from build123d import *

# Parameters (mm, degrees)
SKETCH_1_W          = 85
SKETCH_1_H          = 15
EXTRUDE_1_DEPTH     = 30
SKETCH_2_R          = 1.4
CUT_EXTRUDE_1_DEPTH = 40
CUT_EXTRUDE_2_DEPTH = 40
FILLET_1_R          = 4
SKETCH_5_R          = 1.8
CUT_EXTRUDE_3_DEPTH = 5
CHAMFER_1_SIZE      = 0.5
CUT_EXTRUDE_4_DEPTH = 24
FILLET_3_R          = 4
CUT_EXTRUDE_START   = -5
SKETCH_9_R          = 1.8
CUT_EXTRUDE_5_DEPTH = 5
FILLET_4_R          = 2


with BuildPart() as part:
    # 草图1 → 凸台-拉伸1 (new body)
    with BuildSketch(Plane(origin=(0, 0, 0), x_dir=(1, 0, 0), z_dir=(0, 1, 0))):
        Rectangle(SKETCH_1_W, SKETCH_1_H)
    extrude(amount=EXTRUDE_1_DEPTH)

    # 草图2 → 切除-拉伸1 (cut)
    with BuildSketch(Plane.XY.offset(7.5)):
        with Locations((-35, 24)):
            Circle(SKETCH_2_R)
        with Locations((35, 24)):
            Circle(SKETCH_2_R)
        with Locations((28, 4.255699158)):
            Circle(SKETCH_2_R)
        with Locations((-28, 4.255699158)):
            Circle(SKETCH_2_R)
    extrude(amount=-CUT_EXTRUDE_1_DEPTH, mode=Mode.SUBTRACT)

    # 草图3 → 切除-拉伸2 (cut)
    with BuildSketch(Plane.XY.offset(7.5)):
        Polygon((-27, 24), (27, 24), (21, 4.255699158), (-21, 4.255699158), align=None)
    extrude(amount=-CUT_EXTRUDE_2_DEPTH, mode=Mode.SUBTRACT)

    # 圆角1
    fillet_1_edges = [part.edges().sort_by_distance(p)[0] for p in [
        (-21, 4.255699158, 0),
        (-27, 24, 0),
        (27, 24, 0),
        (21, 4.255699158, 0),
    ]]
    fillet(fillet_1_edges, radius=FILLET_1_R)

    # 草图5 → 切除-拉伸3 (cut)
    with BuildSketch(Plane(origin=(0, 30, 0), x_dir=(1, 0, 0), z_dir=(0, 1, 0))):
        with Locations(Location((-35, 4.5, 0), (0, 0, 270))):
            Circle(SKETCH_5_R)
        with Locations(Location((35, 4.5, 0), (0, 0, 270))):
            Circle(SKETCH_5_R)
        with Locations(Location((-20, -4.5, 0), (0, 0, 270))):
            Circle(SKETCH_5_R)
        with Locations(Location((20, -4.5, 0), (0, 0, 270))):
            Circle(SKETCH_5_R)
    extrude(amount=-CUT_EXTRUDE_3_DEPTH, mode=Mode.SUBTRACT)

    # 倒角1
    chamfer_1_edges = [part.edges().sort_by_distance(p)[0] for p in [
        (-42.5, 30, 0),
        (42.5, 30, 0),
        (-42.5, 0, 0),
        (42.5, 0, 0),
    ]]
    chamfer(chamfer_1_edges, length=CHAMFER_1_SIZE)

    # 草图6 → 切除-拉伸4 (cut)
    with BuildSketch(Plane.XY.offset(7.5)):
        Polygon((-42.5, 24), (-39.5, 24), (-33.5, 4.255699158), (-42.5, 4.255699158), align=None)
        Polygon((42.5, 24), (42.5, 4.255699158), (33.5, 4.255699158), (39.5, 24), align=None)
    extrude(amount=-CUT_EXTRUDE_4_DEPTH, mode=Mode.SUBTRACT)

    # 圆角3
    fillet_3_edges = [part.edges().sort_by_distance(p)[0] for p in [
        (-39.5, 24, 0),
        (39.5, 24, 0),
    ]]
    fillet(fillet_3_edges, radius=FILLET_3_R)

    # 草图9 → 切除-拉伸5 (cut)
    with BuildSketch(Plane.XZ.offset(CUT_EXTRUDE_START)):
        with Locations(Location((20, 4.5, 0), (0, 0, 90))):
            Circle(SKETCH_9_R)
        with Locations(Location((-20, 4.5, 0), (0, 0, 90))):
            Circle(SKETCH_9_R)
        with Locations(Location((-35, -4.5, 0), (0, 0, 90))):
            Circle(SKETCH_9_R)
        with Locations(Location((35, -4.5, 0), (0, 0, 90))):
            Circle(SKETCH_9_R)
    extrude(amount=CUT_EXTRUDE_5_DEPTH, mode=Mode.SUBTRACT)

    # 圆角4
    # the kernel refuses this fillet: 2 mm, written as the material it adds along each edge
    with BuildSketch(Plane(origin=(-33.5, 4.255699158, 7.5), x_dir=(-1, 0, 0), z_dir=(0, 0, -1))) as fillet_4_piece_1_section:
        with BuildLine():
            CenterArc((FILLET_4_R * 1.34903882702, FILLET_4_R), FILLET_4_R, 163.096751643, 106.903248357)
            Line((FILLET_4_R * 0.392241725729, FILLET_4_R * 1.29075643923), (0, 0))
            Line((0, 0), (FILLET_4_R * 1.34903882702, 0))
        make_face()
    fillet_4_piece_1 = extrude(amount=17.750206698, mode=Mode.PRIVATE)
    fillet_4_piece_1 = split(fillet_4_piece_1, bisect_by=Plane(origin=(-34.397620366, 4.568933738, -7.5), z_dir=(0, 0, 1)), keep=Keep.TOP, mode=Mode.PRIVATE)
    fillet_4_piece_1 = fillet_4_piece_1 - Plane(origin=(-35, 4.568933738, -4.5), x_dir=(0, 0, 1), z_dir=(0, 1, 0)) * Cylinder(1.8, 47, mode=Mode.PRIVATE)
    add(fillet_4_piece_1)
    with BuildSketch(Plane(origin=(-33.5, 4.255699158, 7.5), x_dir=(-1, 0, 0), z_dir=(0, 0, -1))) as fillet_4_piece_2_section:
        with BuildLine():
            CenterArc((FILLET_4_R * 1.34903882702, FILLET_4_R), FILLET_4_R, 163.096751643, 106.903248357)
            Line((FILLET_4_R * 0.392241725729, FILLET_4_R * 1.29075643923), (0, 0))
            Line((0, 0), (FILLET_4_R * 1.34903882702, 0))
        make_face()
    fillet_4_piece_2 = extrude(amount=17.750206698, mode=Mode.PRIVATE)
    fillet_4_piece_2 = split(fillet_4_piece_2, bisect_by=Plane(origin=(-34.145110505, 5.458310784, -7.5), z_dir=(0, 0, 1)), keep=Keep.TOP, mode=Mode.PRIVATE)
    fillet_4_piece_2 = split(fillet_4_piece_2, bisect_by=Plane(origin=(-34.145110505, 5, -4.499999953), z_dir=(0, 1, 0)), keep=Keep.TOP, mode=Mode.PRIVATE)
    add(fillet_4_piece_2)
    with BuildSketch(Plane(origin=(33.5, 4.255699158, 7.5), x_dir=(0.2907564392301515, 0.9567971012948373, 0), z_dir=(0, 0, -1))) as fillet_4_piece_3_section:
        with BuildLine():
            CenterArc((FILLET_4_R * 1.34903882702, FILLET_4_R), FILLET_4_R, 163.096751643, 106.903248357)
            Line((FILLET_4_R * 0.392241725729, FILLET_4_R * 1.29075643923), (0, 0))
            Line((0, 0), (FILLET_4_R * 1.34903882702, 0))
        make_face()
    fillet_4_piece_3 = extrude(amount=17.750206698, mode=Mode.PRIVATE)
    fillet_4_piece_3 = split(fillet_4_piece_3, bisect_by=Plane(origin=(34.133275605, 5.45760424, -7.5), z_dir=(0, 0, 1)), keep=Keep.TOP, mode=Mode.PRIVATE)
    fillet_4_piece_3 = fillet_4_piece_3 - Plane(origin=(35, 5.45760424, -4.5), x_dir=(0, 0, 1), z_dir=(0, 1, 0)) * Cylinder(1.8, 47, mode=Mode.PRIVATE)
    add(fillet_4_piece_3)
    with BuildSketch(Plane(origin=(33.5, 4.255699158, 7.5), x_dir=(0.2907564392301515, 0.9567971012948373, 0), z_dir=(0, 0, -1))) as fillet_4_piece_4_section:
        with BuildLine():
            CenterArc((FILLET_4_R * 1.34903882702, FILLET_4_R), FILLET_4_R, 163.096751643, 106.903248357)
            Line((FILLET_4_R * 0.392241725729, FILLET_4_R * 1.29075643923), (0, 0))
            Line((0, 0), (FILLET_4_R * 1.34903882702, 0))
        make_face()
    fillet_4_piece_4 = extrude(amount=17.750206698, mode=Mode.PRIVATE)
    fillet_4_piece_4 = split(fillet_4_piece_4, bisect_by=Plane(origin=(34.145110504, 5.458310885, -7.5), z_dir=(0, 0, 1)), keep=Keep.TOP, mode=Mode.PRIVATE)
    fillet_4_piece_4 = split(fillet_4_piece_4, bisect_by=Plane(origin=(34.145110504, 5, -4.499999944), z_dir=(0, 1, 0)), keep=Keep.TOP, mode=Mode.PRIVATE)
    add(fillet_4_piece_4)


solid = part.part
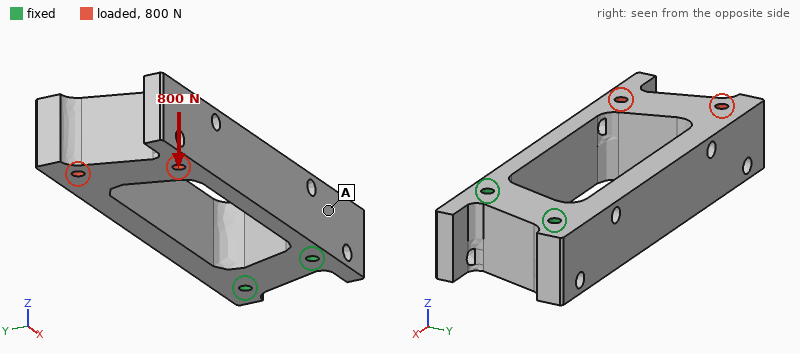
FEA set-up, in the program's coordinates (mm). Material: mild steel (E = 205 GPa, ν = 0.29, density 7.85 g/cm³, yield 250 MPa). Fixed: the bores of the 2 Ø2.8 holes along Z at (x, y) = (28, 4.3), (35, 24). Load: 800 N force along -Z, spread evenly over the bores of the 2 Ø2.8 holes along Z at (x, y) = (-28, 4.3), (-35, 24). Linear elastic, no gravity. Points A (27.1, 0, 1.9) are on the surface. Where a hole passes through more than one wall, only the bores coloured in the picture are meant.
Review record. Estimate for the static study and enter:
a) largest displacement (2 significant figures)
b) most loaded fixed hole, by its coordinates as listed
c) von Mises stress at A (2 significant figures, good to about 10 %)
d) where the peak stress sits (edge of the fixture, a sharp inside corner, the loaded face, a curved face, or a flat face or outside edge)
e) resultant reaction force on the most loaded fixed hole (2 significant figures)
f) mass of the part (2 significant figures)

0.15 mm
(28, 4.3)
23 MPa
a curved face
660 N
160 g
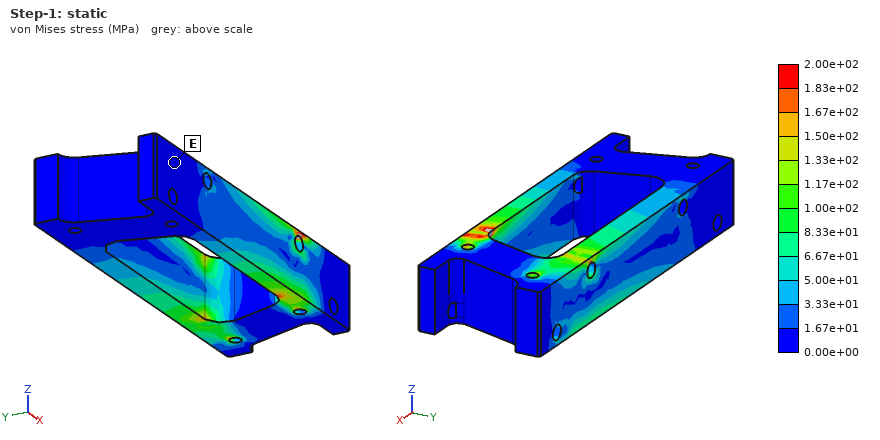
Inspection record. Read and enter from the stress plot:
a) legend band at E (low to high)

0.00e+00 to 1.67e+01 MPa
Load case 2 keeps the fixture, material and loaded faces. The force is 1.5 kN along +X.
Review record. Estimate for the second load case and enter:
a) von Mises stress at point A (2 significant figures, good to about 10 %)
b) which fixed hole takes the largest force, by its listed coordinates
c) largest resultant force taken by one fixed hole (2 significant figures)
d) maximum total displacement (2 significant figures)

7.3 MPa
(28, 4.3)
810 N
5.0 µm
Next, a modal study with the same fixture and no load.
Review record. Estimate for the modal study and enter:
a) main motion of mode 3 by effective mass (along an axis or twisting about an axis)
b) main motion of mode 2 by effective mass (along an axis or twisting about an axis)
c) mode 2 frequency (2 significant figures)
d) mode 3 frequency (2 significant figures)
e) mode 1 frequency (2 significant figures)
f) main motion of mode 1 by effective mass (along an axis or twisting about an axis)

twisting about X
along Z
1700 Hz
4100 Hz
1400 Hz
along Y
